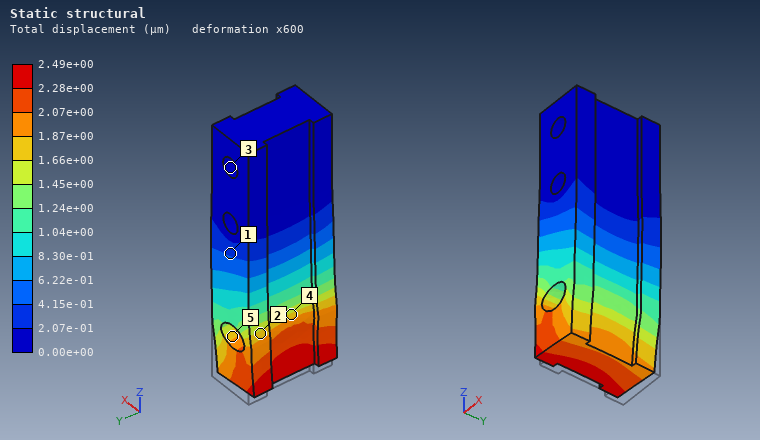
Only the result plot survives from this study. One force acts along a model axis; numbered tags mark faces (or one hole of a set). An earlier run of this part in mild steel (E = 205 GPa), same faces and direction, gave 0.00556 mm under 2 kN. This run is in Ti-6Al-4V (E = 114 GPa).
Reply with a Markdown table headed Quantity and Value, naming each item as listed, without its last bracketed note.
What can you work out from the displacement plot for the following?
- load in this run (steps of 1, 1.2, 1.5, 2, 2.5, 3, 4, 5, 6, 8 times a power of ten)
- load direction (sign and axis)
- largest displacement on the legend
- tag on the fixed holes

| Quantity | Value |
|---|---|
| load in this run | 500 N |
| load direction | +Z |
| largest displacement on the legend | 2.49e+00 µm |
| tag on the fixed holes | 3 |
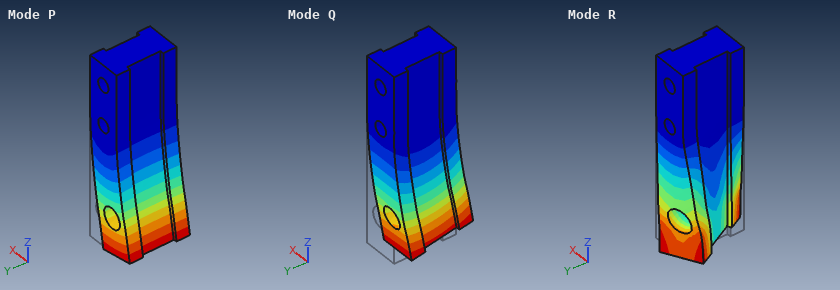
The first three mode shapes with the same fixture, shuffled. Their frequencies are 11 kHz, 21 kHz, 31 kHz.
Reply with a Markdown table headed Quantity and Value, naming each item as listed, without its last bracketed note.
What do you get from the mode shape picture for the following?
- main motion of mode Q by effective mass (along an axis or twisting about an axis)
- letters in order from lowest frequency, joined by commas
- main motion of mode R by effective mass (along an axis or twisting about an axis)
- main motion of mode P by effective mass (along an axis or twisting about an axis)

| Quantity | Value |
|---|---|
| main motion of mode Q by effective mass | along Y |
| letters in order from lowest frequency, joined by commas | P, Q, R |
| main motion of mode R by effective mass | twisting about Z |
| main motion of mode P by effective mass | along X |
